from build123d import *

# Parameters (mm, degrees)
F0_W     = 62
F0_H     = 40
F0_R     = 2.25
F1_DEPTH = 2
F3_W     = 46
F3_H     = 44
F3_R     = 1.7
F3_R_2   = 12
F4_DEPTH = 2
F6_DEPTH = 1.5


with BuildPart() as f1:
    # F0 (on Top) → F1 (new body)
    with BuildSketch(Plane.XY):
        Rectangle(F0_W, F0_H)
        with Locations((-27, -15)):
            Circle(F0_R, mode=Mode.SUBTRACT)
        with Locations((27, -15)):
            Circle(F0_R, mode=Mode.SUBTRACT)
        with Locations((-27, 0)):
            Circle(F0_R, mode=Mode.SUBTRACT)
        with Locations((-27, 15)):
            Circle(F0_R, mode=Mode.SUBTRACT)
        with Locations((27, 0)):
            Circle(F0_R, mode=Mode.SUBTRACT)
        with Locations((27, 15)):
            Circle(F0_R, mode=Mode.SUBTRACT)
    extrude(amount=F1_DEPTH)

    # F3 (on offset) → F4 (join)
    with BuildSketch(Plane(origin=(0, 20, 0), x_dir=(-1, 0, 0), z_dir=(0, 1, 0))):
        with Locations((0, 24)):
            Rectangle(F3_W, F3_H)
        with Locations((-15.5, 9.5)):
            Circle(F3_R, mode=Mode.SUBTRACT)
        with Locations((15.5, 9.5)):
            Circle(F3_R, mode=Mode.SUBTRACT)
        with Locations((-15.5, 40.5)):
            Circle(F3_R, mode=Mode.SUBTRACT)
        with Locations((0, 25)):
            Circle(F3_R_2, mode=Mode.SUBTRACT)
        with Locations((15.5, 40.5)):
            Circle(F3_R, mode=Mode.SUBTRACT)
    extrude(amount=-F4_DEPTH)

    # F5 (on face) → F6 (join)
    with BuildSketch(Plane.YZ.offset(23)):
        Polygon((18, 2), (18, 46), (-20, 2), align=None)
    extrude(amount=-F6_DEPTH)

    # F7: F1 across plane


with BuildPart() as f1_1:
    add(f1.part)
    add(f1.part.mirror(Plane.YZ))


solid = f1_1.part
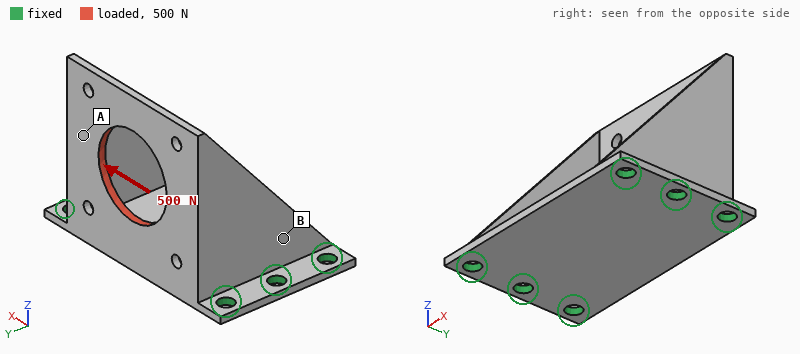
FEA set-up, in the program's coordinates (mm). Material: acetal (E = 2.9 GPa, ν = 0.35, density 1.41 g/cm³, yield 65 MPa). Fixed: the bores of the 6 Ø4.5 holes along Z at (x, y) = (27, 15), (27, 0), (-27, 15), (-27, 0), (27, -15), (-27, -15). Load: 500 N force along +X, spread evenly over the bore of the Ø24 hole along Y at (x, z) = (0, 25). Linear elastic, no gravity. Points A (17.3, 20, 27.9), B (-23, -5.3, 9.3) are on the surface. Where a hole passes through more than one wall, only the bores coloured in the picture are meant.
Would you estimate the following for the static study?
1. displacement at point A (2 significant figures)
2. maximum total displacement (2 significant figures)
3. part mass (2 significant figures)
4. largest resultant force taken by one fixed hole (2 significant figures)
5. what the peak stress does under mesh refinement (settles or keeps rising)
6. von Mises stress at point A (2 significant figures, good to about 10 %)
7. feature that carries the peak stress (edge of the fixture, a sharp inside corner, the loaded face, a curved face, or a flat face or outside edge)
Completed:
0.52 mm
0.84 mm
15 g
320 N
keeps rising
8.5 MPa
edge of the fixture
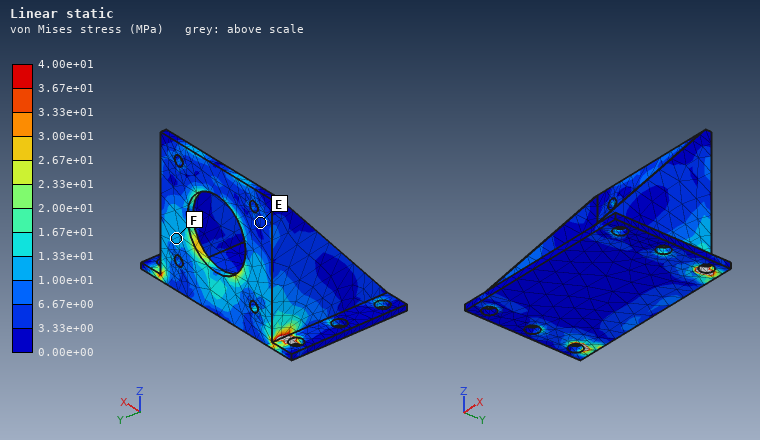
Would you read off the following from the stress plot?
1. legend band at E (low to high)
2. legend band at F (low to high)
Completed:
3.33e+00 to 6.67e+00 MPa
1.00e+01 to 1.33e+01 MPa
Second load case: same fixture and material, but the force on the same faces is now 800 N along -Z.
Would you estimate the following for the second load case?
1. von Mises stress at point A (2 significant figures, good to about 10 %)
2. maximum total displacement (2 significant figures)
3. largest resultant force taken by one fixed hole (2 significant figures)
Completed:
12 MPa
0.88 mm
440 N
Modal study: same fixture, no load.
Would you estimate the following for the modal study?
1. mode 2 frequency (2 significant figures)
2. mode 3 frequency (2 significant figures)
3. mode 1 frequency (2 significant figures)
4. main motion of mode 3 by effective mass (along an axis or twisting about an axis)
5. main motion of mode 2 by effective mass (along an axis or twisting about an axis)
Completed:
1300 Hz
1400 Hz
830 Hz
along X
along Z
